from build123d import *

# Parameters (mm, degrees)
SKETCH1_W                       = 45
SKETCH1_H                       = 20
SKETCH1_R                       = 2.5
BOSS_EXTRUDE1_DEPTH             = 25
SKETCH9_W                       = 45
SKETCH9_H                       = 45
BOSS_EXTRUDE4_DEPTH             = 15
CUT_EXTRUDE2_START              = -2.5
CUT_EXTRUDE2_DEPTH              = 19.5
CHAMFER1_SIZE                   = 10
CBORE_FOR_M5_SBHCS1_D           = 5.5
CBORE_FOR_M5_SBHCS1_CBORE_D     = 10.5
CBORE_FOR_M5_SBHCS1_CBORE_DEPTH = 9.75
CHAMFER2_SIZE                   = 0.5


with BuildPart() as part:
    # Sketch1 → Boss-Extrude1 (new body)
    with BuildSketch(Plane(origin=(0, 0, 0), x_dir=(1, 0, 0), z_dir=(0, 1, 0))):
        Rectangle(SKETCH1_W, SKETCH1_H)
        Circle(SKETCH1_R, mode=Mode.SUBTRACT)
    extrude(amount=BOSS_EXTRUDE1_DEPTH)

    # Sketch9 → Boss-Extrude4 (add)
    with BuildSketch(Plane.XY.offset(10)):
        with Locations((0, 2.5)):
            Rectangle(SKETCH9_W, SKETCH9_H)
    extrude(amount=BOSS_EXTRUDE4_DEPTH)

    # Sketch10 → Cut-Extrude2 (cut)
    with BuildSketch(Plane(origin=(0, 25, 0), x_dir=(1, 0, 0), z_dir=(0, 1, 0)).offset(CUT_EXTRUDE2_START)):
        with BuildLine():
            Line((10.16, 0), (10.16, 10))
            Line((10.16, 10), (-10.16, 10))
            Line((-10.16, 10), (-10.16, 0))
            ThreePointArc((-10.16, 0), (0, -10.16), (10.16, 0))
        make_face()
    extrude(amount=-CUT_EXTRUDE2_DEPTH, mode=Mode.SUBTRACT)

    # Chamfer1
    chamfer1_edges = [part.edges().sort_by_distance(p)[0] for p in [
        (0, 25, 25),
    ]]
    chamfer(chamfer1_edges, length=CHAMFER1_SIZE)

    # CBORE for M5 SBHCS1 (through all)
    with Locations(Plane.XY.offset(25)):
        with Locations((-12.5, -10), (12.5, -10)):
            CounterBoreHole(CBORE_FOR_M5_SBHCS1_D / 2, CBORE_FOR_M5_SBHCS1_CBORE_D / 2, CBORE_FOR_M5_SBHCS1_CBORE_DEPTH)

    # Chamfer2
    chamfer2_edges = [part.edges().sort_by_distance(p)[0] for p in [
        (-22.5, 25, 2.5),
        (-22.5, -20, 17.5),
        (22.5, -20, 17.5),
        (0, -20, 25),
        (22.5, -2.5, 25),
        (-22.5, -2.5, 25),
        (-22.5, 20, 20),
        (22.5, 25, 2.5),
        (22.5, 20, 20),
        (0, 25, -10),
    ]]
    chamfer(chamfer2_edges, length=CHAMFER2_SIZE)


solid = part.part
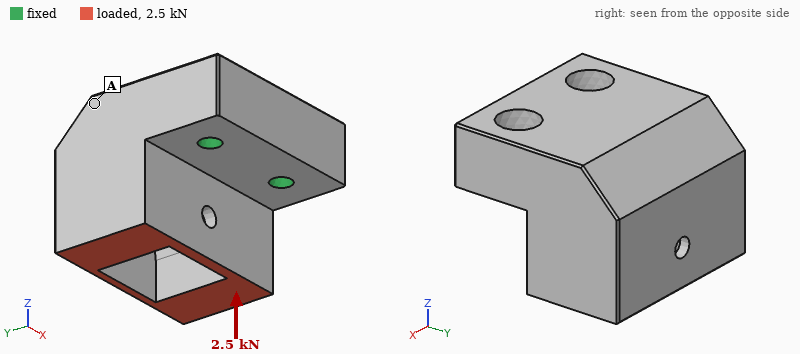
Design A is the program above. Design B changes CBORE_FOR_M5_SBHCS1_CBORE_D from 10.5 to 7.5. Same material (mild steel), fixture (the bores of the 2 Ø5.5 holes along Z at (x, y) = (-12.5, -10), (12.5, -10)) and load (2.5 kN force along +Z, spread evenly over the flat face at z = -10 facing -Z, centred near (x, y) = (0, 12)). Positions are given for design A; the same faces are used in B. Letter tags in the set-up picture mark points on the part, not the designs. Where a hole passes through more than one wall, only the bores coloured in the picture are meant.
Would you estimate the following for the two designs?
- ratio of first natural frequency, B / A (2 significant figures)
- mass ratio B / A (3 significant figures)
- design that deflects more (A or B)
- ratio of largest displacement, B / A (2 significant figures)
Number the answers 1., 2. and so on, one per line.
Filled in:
1. 1.1
2. 1.02
3. A
4. 0.90
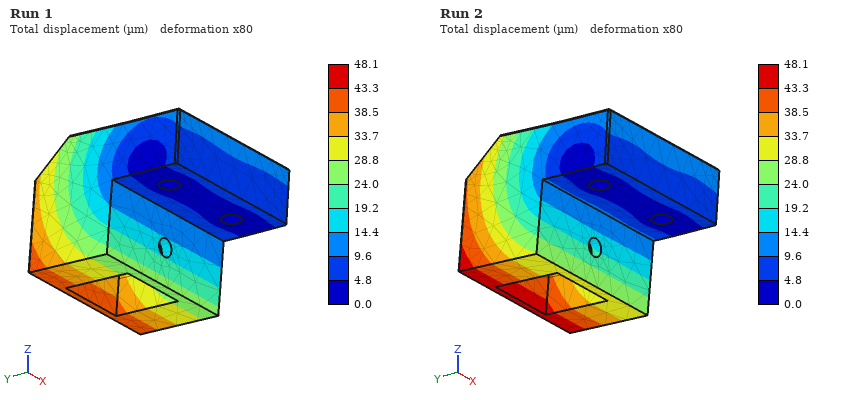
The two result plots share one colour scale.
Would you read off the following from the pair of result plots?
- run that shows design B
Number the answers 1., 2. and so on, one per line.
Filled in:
1. Run 1
